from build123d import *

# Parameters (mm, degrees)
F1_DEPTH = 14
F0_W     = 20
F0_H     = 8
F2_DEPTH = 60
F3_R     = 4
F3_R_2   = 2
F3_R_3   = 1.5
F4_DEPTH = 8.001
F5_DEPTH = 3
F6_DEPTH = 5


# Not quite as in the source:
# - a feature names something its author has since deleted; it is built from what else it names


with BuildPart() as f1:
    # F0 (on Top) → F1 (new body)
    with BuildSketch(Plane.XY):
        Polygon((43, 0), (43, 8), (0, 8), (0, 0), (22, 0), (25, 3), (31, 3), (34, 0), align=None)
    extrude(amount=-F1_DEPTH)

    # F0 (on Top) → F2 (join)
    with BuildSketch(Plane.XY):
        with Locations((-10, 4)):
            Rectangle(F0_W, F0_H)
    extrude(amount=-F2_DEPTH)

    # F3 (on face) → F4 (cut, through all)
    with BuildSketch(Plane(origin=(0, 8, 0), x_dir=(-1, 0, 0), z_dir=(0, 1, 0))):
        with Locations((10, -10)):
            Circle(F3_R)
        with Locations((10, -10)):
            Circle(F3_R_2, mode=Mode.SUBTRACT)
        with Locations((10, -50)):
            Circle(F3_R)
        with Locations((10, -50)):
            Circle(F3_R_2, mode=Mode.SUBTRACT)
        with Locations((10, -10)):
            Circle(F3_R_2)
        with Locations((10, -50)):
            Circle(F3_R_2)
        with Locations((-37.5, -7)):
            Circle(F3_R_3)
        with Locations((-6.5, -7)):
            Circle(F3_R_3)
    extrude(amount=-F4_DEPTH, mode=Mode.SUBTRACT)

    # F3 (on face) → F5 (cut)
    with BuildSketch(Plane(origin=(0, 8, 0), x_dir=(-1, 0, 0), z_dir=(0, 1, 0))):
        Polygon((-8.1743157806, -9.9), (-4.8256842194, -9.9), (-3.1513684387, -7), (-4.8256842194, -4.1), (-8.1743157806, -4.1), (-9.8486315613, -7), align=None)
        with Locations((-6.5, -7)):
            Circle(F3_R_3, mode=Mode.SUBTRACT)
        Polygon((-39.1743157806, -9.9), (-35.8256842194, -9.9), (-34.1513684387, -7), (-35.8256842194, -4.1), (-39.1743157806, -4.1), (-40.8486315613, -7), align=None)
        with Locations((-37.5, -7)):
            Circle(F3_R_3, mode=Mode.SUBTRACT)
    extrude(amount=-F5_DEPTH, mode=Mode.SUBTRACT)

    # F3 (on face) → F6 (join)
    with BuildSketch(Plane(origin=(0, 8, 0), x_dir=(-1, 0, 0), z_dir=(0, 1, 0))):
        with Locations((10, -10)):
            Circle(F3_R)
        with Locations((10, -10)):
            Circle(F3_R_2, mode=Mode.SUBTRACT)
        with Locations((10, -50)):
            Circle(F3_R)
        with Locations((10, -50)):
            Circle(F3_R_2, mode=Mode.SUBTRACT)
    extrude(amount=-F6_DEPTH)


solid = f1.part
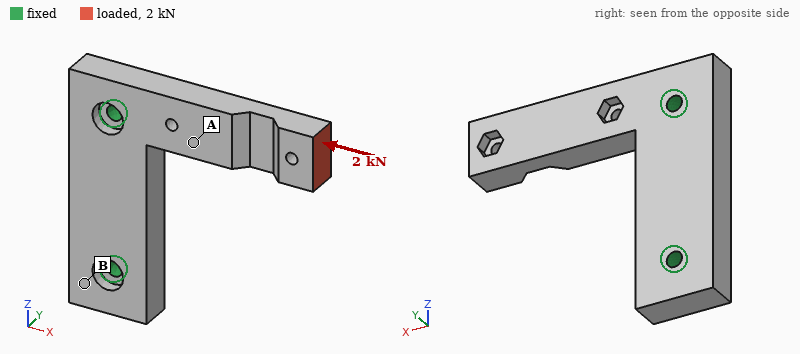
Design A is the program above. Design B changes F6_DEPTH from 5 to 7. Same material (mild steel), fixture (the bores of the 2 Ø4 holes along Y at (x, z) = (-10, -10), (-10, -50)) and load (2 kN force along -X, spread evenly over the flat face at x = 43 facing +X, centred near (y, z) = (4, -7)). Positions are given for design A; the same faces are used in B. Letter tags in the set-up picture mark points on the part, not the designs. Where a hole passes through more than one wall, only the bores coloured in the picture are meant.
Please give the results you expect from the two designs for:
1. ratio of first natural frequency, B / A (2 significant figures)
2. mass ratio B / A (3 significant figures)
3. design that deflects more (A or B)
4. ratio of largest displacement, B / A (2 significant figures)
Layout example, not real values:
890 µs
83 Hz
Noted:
1.1
1.01
A
0.72
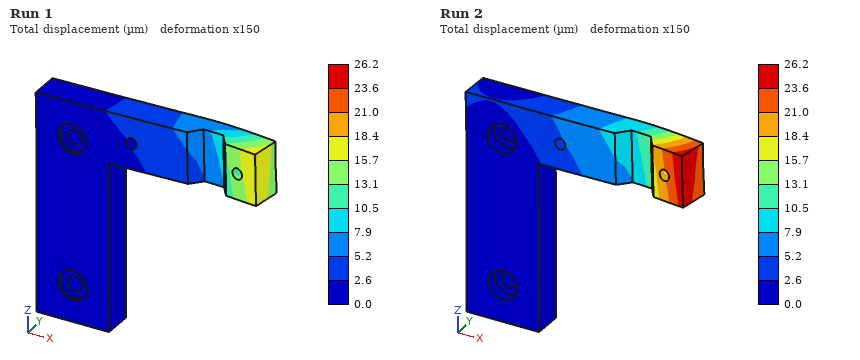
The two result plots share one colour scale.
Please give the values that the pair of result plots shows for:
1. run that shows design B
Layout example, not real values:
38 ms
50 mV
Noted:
Run 1
